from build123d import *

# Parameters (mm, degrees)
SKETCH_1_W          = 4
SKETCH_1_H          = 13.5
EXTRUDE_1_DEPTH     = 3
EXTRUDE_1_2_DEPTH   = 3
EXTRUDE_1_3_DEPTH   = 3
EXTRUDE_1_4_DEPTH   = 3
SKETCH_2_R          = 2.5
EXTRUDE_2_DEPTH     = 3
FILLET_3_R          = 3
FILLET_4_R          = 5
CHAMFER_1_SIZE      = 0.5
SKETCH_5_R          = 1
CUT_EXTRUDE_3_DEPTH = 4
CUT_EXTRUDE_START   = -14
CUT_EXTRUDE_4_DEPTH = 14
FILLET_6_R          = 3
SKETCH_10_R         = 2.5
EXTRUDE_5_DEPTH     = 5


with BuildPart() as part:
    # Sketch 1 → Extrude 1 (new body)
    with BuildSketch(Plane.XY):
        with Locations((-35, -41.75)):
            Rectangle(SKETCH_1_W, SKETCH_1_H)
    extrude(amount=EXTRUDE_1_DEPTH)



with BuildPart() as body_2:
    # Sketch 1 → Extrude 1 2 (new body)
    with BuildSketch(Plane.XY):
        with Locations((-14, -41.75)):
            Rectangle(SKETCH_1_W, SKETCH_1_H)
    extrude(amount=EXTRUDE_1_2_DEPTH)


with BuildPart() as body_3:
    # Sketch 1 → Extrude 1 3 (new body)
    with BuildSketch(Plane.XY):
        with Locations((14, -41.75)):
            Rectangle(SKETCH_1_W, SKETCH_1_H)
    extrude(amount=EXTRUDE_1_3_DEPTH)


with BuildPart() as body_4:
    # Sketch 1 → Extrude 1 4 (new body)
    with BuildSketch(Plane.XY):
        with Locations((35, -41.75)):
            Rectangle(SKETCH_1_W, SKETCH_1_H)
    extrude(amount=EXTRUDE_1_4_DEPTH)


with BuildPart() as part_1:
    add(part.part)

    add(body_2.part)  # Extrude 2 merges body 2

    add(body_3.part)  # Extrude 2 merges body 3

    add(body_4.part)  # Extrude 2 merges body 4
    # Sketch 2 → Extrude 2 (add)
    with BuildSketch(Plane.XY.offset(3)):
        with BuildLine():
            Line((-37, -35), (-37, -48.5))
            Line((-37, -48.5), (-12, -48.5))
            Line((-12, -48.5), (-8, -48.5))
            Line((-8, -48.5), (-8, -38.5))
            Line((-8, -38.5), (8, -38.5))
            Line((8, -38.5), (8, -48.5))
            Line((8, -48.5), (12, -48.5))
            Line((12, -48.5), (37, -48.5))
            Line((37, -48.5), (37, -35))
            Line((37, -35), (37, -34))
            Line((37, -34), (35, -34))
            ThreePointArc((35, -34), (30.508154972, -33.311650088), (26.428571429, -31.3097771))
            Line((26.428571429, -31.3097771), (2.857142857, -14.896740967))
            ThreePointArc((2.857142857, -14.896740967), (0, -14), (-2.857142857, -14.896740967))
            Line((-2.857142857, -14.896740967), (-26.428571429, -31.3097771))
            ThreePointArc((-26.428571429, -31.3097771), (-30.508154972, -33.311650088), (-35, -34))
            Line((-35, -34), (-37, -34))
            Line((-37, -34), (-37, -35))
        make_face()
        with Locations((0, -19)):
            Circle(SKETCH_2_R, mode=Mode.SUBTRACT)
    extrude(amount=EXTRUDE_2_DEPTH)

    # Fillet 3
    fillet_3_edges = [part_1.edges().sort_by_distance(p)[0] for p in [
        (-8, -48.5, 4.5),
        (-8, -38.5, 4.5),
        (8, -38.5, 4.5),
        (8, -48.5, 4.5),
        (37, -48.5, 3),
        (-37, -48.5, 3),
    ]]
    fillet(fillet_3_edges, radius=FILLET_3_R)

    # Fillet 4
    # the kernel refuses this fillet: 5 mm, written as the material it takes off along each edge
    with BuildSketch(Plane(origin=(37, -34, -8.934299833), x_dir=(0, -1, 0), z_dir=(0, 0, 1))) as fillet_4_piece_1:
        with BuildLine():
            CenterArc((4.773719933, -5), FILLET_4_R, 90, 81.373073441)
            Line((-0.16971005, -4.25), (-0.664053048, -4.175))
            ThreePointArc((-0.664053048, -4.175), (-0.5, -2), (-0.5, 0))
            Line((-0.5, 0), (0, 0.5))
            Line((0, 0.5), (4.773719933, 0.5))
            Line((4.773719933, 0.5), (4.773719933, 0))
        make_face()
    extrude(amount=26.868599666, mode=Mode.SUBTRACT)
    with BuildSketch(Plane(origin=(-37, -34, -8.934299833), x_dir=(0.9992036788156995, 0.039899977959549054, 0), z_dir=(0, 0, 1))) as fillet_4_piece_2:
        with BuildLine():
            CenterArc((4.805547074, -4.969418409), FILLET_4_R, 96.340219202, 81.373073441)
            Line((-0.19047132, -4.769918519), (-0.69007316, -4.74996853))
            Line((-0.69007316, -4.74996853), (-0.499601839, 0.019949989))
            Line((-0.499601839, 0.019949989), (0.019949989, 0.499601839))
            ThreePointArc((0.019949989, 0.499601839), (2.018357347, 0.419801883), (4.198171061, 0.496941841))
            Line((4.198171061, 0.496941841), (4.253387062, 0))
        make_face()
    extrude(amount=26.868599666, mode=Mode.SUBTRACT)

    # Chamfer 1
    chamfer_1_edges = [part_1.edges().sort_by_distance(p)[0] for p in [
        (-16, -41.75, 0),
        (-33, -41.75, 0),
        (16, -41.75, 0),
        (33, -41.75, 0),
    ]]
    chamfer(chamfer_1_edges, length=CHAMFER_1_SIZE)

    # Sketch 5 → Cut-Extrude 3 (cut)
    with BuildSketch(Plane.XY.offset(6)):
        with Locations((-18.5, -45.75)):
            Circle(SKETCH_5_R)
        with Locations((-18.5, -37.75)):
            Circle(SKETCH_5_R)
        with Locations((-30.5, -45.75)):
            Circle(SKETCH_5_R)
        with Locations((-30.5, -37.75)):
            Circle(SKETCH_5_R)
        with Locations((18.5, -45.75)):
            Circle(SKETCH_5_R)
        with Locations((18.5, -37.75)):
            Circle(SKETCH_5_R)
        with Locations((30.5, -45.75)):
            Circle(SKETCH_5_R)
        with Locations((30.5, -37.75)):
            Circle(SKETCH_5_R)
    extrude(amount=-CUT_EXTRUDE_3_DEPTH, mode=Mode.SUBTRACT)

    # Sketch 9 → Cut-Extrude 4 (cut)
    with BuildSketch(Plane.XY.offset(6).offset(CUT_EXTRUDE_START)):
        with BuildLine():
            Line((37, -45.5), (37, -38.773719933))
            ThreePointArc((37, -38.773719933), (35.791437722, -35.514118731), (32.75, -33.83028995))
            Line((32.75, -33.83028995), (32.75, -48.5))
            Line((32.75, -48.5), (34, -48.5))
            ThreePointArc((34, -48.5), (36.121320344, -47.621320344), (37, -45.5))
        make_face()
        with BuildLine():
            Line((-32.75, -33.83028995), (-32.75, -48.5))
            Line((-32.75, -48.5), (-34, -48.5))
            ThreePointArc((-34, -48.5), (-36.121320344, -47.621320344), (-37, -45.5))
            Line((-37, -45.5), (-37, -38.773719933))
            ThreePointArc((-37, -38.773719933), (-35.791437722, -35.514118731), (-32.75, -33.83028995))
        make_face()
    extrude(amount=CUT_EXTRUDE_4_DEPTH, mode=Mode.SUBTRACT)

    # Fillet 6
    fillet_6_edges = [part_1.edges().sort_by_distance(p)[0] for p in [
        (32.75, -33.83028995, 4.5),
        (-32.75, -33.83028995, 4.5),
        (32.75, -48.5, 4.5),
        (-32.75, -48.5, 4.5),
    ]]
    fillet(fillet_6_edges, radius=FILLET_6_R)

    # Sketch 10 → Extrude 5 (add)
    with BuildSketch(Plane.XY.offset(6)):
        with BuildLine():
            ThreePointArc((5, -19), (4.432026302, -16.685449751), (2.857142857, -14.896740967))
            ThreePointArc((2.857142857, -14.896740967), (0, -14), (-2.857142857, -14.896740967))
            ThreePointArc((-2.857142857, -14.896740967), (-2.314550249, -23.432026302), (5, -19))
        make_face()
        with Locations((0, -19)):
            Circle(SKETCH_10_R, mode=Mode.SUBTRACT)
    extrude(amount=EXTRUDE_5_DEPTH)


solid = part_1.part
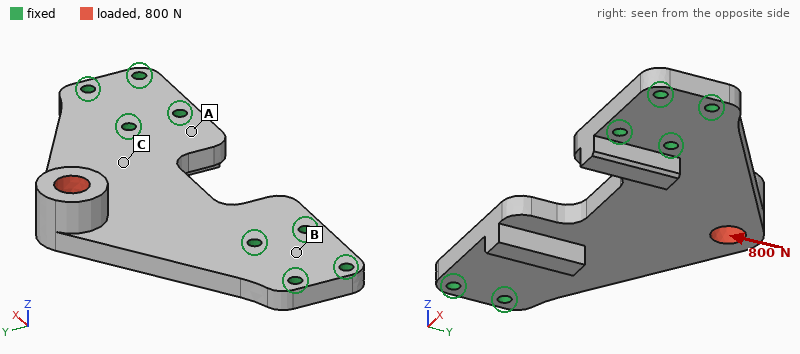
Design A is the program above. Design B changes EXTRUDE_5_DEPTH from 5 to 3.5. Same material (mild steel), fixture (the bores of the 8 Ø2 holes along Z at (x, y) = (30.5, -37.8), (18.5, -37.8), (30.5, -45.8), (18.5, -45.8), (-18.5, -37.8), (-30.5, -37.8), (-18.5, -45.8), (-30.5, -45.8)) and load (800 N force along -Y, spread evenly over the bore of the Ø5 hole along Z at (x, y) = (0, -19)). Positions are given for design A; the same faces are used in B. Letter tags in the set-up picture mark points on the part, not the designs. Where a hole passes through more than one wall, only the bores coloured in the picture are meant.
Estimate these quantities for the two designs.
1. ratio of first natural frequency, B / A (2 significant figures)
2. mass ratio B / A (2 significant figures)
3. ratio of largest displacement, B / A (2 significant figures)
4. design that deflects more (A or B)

1.1
0.98
0.70
A
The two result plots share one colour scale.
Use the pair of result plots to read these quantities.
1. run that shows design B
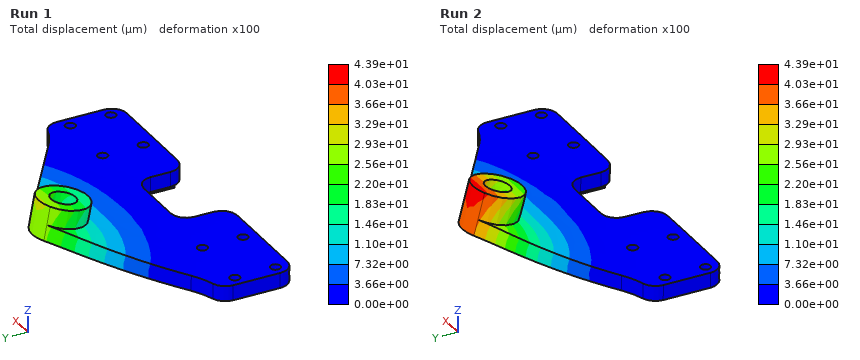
Run 1
